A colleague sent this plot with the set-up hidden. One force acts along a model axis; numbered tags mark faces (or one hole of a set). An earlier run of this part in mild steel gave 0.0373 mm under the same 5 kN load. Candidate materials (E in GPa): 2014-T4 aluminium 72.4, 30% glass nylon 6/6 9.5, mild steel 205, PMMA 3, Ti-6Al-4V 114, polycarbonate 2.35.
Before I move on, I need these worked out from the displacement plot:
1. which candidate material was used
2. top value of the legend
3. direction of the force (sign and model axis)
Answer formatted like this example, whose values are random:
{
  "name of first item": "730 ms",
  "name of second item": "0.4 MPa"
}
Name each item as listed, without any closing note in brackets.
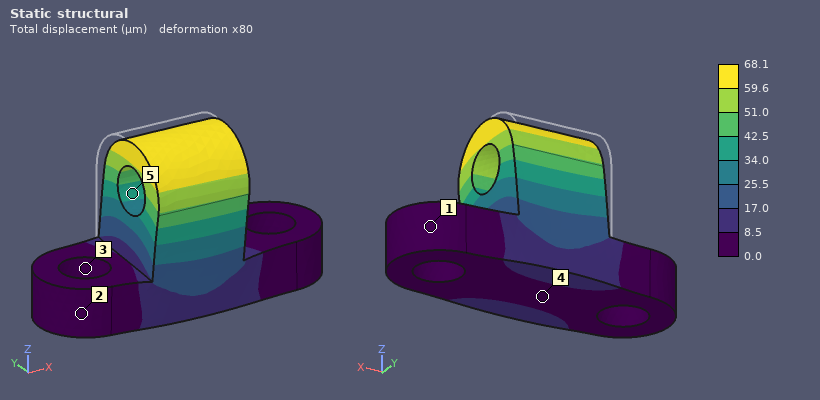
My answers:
{
  "which candidate material was used": "Ti-6Al-4V",
  "top value of the legend": "68.1 µm",
  "direction of the force": "-Y"
}
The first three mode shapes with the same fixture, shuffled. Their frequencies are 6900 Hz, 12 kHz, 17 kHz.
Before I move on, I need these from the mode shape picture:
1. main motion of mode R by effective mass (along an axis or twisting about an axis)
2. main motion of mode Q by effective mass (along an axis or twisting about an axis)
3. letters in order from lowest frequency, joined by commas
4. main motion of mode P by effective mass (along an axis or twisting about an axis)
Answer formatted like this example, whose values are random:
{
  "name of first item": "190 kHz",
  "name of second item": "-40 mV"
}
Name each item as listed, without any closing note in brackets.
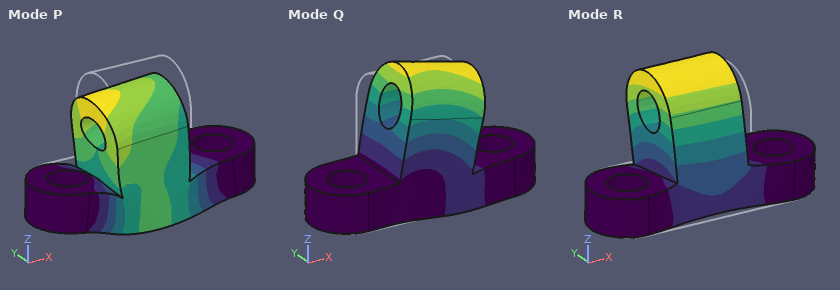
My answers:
{
  "main motion of mode R by effective mass": "along Y",
  "main motion of mode Q by effective mass": "along X",
  "letters in order from lowest frequency, joined by commas": "R, Q, P",
  "main motion of mode P by effective mass": "along Z"
}
